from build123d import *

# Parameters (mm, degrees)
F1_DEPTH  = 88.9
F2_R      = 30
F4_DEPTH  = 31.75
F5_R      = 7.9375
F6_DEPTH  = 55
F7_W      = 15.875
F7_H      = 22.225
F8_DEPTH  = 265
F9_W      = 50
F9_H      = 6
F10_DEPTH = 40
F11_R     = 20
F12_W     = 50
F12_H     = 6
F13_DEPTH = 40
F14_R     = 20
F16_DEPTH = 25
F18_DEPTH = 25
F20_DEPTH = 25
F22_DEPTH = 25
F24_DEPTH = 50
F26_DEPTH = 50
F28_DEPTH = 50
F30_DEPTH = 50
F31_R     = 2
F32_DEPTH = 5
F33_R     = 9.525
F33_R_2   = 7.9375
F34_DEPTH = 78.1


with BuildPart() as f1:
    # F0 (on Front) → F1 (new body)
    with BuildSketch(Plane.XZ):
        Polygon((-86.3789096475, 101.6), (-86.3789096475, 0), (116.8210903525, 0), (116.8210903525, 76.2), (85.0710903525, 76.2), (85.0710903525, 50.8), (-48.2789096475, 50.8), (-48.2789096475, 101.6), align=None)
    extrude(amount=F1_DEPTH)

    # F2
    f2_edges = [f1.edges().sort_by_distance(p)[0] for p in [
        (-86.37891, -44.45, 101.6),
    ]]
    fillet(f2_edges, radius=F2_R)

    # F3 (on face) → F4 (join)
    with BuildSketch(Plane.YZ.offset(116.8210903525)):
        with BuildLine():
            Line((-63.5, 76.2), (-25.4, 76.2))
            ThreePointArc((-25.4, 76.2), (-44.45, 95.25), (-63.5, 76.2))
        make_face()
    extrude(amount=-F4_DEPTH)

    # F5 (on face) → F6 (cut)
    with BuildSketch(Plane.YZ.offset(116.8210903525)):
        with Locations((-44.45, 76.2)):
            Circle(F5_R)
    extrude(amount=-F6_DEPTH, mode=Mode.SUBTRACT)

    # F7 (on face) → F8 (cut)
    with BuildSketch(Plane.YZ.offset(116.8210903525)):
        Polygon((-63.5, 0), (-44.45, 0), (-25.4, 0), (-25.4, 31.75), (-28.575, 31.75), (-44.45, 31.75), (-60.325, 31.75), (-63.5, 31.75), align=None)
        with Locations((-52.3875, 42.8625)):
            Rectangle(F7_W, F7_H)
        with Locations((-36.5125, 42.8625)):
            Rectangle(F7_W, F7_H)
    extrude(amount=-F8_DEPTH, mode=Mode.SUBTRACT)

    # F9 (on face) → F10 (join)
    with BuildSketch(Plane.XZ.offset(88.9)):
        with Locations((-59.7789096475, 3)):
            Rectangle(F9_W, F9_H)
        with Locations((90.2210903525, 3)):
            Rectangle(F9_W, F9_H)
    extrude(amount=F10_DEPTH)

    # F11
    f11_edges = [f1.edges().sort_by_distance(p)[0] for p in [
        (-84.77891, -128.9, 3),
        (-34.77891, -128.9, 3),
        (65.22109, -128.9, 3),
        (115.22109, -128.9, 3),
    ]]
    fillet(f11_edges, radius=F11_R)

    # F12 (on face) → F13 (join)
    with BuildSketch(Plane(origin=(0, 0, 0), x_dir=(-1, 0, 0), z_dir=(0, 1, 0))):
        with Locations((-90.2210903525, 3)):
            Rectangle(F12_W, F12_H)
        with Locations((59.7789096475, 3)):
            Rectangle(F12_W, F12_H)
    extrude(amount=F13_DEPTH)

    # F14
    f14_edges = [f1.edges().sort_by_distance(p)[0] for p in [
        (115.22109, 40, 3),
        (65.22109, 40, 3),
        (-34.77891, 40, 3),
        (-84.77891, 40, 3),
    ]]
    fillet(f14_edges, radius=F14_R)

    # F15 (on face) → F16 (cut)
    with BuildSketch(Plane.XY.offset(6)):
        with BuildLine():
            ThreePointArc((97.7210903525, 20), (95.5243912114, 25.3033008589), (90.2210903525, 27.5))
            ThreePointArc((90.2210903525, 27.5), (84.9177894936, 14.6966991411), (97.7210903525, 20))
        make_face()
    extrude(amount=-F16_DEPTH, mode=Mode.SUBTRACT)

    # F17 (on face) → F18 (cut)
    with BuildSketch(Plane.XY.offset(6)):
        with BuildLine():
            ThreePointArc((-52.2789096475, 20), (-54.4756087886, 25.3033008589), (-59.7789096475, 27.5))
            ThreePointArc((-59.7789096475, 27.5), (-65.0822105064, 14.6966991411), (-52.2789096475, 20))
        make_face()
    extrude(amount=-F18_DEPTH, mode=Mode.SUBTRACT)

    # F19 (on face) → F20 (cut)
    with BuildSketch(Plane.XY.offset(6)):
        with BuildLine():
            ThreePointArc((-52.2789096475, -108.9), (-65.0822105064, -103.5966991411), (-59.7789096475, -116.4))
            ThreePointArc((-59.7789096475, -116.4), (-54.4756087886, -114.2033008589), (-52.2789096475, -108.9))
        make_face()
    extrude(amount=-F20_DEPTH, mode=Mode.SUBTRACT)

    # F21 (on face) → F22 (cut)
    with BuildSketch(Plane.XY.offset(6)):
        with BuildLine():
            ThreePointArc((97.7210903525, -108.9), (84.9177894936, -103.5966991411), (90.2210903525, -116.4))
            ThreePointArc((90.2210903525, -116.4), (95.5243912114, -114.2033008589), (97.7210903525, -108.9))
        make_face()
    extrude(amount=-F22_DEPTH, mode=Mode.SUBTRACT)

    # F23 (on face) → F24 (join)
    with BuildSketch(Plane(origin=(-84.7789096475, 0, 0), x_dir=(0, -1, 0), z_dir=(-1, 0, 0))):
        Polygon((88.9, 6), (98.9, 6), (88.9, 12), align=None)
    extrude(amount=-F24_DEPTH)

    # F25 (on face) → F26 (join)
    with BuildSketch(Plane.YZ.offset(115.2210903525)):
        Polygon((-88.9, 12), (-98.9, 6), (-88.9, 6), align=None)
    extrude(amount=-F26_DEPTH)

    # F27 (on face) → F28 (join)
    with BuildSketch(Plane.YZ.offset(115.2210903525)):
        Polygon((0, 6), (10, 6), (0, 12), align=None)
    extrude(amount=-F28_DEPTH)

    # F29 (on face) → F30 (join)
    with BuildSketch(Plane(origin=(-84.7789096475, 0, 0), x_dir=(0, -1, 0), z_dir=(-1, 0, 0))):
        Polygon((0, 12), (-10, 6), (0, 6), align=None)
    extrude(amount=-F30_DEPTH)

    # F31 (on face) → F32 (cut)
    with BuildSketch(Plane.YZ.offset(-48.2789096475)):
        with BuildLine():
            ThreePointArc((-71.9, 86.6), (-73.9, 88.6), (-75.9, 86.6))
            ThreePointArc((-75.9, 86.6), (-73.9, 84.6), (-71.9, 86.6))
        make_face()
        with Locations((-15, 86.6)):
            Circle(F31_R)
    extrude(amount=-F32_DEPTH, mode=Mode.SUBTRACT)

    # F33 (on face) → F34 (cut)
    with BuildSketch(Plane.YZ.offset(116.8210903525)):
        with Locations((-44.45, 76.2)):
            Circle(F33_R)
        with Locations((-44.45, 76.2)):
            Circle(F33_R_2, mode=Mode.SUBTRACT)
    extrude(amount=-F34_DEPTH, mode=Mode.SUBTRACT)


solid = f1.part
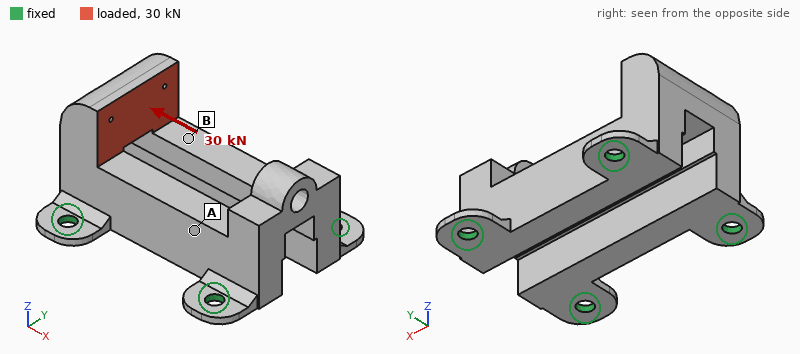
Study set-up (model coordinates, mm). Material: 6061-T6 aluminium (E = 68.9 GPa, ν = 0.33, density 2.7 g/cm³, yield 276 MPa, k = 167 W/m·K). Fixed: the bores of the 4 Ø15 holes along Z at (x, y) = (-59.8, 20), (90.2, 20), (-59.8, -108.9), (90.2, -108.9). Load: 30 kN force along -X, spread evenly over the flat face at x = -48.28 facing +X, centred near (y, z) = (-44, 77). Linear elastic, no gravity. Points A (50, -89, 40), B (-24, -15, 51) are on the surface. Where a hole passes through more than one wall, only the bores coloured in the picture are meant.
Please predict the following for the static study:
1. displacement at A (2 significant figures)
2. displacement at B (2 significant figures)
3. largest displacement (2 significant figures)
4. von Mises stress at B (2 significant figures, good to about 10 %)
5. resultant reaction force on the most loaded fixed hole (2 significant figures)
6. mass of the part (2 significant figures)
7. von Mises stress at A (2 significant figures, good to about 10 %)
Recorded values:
0.082 mm
0.10 mm
0.35 mm
55 MPa
13 kN
2.2 kg
26 MPa
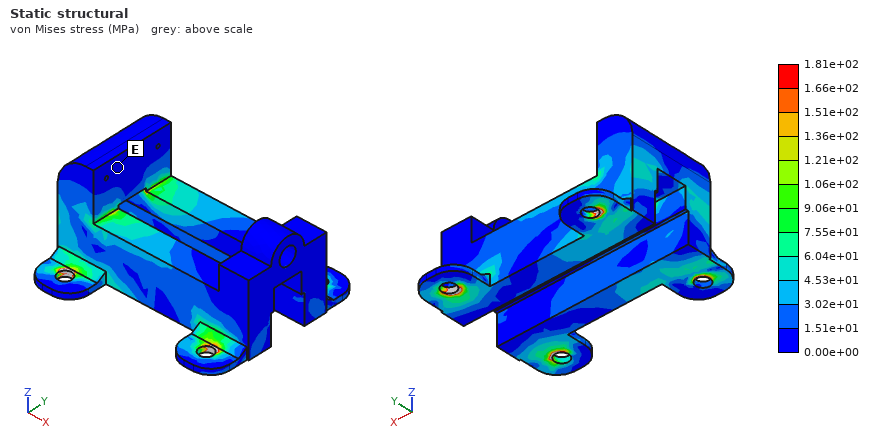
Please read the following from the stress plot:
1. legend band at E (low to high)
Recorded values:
0.00e+00 to 1.51e+01 MPa
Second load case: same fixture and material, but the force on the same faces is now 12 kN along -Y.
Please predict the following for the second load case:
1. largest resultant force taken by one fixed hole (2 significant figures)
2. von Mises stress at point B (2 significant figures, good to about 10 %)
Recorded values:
9.0 kN
11 MPa
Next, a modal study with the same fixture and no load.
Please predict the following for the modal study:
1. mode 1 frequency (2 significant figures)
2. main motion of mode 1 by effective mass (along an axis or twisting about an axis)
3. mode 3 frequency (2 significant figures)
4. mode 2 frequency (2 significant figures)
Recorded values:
2000 Hz
along X
2400 Hz
2300 Hz
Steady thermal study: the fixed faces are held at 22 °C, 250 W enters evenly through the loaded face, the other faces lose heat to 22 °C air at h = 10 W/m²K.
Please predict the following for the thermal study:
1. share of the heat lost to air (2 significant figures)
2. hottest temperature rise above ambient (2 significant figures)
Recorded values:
10 %
69 K
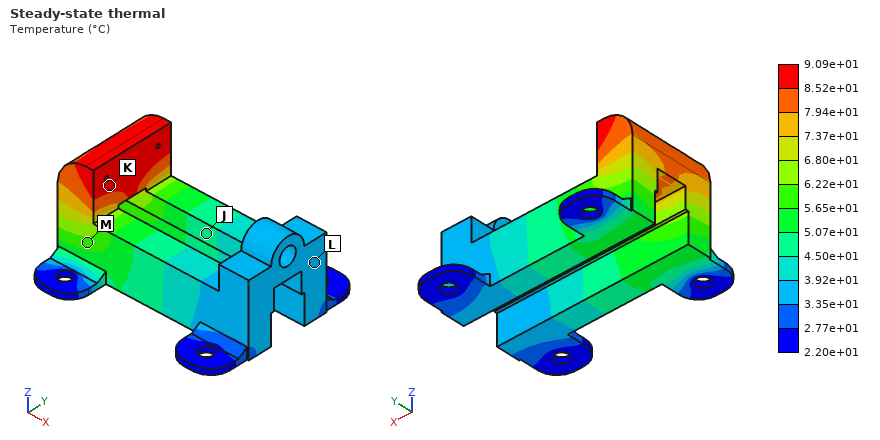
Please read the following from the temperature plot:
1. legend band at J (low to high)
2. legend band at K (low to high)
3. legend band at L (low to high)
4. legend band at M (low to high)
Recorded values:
4.50e+01 to 5.07e+01 °C
8.52e+01 to 9.09e+01 °C
3.35e+01 to 3.92e+01 °C
5.65e+01 to 6.22e+01 °C
